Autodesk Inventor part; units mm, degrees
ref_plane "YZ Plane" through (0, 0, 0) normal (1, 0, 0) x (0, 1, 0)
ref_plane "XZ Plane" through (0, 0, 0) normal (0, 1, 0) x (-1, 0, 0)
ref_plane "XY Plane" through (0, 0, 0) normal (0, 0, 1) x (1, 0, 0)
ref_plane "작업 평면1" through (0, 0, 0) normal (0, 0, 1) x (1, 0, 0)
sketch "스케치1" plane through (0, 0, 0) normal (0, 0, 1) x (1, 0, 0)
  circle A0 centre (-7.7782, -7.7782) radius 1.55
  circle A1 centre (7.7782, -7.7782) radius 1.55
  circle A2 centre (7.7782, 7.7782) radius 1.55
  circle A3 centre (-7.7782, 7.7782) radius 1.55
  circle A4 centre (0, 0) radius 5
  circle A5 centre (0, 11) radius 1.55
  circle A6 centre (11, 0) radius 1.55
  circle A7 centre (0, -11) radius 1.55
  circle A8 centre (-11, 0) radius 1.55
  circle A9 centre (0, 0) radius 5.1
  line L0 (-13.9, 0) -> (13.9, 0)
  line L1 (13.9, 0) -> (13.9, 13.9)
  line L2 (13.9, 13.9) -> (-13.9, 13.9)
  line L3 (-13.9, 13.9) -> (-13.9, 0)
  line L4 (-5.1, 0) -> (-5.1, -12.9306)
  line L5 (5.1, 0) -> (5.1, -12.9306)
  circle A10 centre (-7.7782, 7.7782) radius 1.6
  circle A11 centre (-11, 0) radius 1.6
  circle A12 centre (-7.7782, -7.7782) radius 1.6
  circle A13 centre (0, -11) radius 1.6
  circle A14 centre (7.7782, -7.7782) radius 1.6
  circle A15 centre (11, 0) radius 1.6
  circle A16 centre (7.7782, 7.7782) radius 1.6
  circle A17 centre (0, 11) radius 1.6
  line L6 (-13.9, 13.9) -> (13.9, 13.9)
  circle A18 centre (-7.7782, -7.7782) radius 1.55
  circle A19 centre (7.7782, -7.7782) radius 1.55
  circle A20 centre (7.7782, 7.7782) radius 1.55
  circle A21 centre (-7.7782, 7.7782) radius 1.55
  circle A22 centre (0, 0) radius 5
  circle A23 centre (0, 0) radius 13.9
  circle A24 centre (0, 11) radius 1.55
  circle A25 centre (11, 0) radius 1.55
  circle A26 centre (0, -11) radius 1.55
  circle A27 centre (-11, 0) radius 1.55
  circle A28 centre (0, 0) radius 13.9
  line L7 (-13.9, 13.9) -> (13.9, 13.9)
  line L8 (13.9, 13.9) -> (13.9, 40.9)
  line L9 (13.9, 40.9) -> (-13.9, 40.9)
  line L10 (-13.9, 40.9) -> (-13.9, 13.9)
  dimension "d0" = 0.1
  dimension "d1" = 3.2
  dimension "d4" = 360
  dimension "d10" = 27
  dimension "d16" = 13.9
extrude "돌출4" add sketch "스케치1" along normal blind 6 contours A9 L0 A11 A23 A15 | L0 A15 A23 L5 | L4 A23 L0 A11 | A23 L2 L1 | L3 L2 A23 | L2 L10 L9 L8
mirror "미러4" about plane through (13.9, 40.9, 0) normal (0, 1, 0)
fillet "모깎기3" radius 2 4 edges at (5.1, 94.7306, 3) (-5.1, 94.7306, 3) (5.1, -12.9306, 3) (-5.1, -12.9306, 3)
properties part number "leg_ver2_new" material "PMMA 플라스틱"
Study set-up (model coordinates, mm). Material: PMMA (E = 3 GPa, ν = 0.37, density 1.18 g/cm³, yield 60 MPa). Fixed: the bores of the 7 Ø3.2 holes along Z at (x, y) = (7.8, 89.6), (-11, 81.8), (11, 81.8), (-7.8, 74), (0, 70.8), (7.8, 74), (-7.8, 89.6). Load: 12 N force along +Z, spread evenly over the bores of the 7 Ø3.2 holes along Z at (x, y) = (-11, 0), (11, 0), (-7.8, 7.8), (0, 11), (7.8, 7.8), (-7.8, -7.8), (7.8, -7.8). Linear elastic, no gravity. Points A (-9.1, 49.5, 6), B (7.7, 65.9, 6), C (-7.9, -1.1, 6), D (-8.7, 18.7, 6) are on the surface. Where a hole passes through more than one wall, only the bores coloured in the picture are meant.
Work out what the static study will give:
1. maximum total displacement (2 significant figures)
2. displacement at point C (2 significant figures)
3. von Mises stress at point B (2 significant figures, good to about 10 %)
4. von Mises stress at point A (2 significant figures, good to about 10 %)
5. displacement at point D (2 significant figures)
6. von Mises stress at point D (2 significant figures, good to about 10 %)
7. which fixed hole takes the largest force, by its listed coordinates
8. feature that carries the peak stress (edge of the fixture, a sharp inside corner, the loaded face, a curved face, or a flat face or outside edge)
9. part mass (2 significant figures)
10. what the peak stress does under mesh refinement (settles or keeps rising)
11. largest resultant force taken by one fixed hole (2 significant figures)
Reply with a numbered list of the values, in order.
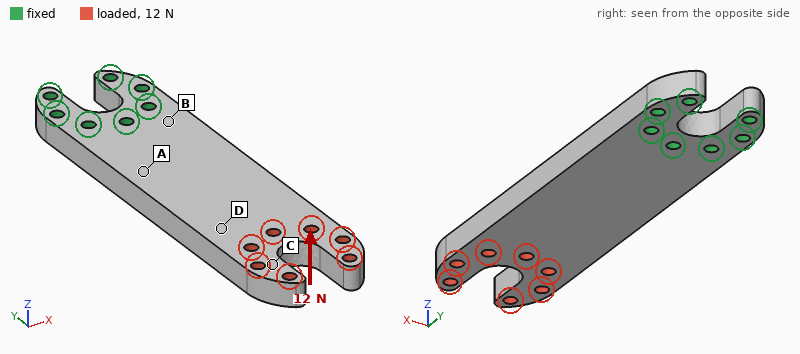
1. 1.2 mm
2. 0.95 mm
3. 4.1 MPa
4. 3.4 MPa
5. 0.57 mm
6. 1.3 MPa
7. (0, 70.8)
8. edge of the fixture
9. 17 g
10. keeps rising
11. 43 N
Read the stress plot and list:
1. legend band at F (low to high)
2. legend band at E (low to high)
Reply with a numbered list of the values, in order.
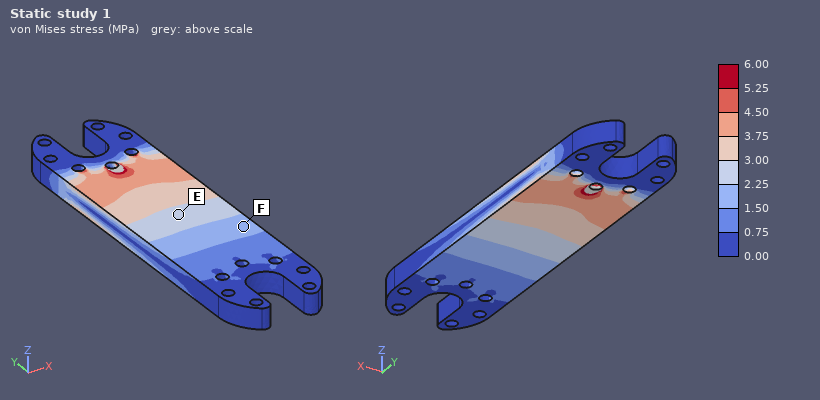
1. 1.50 to 2.25 MPa
2. 2.25 to 3.00 MPa
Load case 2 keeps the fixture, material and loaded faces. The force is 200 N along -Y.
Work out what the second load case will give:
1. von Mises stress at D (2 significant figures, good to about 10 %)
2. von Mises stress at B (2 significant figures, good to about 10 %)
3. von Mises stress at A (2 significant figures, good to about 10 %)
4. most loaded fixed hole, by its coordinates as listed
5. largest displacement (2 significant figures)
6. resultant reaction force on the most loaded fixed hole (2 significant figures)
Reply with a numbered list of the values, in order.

1. 1.2 MPa
2. 1.2 MPa
3. 1.2 MPa
4. (0, 70.8)
5. 34 µm
6. 70 N
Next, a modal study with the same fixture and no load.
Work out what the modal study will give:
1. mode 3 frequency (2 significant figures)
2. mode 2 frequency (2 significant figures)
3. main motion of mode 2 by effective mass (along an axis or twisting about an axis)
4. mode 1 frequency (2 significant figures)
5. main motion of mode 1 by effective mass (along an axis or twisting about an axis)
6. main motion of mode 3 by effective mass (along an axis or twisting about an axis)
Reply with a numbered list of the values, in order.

1. 1300 Hz
2. 1100 Hz
3. along X
4. 280 Hz
5. along Z
6. twisting about Y
